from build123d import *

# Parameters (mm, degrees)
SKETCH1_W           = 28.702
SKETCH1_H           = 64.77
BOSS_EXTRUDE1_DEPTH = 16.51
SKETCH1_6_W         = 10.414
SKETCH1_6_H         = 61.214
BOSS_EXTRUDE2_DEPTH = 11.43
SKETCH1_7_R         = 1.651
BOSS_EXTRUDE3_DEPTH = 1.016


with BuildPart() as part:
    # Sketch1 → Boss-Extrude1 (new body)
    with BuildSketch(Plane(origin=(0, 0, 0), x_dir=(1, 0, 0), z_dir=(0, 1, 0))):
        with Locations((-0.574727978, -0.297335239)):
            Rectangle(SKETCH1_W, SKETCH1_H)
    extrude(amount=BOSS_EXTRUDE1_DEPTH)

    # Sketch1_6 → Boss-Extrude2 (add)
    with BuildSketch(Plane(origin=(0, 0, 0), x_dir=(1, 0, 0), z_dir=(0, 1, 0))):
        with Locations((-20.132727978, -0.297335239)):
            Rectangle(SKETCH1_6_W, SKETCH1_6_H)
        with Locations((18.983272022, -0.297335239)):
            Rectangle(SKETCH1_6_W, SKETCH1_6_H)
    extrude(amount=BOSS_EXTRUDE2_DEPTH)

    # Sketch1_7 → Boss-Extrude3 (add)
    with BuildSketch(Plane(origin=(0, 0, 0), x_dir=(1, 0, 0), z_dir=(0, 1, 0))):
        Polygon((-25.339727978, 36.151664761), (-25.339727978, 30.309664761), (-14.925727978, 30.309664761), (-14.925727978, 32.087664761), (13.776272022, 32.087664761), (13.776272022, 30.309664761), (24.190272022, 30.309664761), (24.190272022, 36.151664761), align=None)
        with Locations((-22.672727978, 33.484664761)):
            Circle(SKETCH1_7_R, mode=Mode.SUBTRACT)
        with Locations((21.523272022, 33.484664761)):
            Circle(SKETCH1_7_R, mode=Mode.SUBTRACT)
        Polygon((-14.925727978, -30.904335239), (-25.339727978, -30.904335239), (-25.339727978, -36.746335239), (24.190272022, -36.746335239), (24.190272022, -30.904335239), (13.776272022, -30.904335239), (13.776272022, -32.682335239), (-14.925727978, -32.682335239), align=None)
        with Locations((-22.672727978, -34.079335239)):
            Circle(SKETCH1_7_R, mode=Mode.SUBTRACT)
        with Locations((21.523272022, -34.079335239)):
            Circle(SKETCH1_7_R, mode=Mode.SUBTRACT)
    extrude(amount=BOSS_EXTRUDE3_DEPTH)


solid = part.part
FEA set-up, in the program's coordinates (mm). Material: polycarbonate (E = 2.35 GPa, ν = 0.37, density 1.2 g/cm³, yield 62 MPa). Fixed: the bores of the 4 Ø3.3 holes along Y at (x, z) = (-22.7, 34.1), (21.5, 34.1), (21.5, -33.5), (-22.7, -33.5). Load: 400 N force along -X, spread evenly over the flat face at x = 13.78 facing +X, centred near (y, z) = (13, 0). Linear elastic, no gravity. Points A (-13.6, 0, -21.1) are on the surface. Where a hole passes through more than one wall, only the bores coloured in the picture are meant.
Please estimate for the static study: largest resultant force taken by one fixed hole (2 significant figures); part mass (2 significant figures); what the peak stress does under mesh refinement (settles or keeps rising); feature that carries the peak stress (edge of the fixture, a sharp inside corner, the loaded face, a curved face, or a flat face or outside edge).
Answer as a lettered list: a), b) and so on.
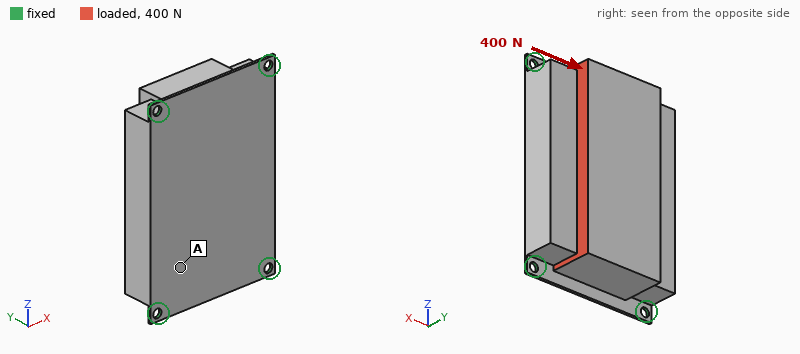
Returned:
a) 130 N
b) 55 g
c) keeps rising
d) edge of the fixture
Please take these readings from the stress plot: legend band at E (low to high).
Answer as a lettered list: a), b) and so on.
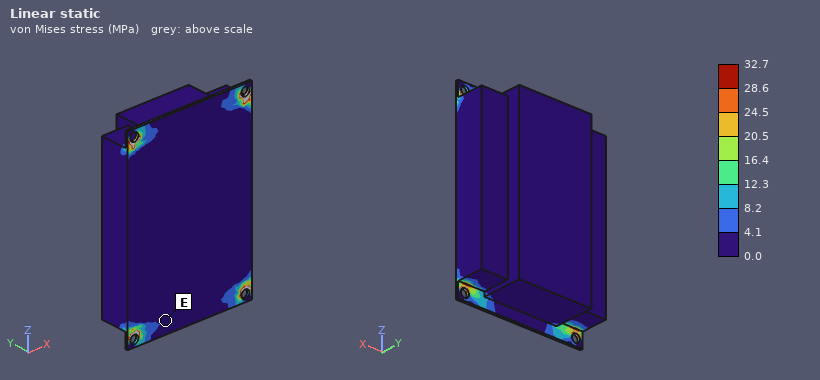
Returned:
a) 0.0 to 4.1 MPa
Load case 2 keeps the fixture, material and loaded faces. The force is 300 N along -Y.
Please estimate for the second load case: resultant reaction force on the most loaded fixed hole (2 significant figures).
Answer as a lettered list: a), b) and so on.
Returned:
a) 150 N
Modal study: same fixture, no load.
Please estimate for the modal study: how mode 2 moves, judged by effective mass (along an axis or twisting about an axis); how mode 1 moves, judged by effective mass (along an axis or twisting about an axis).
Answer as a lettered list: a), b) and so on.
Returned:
a) along X
b) along Y
